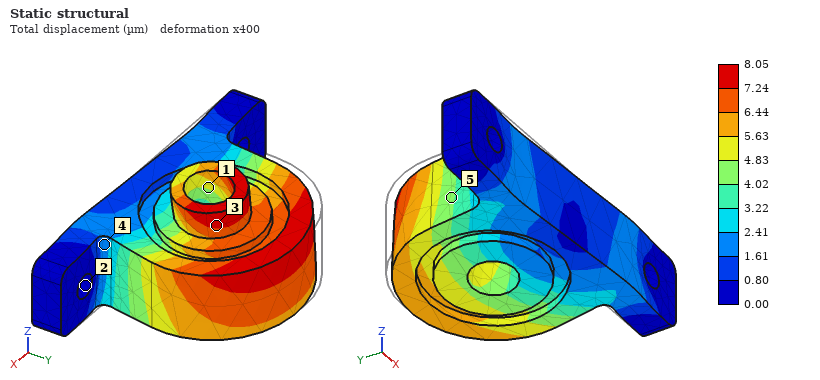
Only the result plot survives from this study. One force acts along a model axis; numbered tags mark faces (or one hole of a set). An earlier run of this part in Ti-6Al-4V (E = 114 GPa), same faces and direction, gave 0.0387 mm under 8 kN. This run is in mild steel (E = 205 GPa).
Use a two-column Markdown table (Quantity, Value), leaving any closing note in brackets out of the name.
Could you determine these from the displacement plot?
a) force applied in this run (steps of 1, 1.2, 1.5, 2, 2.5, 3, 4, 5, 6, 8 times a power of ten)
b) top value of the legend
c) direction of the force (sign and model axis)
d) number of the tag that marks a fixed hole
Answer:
| Quantity | Value |
|---|---|
| force applied in this run | 3 kN |
| top value of the legend | 8.05 µm |
| direction of the force | +X |
| number of the tag that marks a fixed hole | 2 |
